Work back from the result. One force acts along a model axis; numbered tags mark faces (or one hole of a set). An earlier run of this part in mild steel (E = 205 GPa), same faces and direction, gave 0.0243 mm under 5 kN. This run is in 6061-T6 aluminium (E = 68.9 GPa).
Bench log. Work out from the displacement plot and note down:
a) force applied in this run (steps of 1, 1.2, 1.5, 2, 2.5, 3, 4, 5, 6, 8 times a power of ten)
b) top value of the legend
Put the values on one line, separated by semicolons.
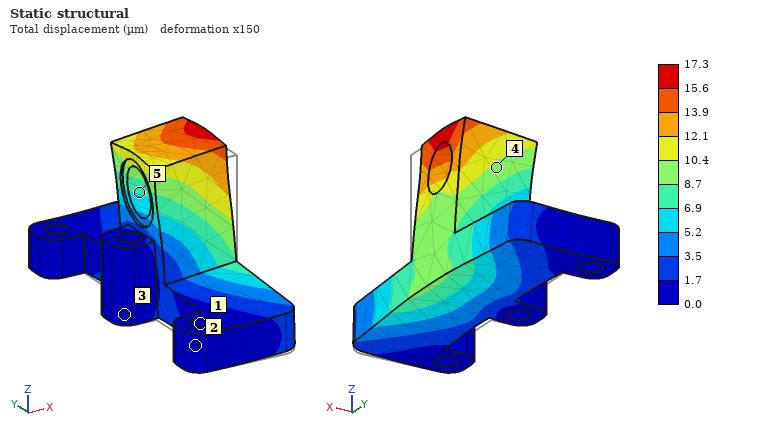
1.2 kN; 17.3 µm
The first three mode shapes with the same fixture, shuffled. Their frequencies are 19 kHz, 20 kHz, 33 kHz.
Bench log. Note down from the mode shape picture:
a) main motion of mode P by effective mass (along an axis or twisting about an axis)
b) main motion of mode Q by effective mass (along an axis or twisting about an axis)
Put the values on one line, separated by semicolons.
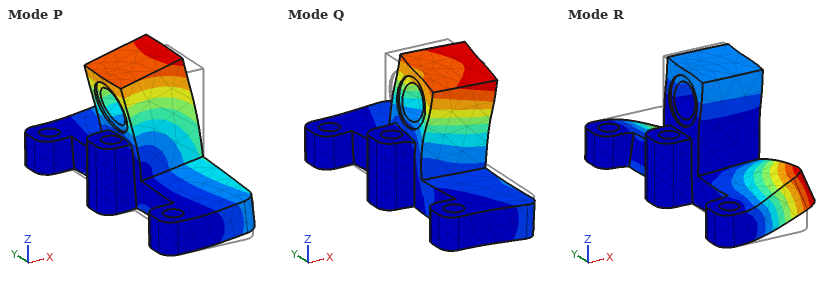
along Z; along Y
